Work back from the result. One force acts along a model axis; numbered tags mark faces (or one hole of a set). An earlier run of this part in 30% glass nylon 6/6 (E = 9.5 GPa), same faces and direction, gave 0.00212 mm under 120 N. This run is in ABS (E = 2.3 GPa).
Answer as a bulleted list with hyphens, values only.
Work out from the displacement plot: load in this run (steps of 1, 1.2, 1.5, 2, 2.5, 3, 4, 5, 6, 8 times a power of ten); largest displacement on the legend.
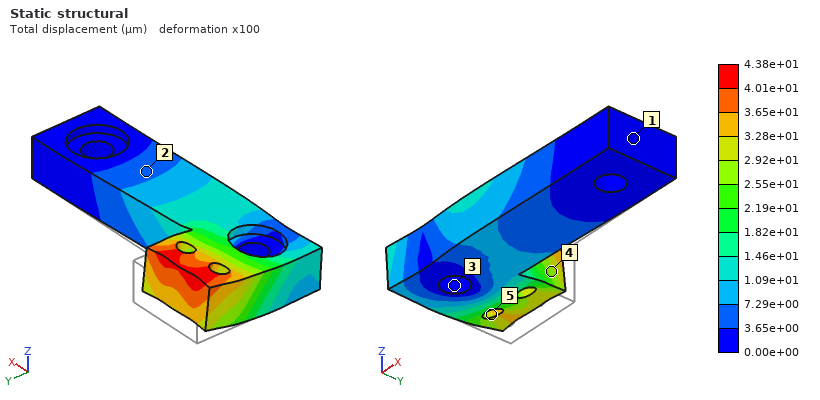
- 600 N
- 4.38e+01 µm
